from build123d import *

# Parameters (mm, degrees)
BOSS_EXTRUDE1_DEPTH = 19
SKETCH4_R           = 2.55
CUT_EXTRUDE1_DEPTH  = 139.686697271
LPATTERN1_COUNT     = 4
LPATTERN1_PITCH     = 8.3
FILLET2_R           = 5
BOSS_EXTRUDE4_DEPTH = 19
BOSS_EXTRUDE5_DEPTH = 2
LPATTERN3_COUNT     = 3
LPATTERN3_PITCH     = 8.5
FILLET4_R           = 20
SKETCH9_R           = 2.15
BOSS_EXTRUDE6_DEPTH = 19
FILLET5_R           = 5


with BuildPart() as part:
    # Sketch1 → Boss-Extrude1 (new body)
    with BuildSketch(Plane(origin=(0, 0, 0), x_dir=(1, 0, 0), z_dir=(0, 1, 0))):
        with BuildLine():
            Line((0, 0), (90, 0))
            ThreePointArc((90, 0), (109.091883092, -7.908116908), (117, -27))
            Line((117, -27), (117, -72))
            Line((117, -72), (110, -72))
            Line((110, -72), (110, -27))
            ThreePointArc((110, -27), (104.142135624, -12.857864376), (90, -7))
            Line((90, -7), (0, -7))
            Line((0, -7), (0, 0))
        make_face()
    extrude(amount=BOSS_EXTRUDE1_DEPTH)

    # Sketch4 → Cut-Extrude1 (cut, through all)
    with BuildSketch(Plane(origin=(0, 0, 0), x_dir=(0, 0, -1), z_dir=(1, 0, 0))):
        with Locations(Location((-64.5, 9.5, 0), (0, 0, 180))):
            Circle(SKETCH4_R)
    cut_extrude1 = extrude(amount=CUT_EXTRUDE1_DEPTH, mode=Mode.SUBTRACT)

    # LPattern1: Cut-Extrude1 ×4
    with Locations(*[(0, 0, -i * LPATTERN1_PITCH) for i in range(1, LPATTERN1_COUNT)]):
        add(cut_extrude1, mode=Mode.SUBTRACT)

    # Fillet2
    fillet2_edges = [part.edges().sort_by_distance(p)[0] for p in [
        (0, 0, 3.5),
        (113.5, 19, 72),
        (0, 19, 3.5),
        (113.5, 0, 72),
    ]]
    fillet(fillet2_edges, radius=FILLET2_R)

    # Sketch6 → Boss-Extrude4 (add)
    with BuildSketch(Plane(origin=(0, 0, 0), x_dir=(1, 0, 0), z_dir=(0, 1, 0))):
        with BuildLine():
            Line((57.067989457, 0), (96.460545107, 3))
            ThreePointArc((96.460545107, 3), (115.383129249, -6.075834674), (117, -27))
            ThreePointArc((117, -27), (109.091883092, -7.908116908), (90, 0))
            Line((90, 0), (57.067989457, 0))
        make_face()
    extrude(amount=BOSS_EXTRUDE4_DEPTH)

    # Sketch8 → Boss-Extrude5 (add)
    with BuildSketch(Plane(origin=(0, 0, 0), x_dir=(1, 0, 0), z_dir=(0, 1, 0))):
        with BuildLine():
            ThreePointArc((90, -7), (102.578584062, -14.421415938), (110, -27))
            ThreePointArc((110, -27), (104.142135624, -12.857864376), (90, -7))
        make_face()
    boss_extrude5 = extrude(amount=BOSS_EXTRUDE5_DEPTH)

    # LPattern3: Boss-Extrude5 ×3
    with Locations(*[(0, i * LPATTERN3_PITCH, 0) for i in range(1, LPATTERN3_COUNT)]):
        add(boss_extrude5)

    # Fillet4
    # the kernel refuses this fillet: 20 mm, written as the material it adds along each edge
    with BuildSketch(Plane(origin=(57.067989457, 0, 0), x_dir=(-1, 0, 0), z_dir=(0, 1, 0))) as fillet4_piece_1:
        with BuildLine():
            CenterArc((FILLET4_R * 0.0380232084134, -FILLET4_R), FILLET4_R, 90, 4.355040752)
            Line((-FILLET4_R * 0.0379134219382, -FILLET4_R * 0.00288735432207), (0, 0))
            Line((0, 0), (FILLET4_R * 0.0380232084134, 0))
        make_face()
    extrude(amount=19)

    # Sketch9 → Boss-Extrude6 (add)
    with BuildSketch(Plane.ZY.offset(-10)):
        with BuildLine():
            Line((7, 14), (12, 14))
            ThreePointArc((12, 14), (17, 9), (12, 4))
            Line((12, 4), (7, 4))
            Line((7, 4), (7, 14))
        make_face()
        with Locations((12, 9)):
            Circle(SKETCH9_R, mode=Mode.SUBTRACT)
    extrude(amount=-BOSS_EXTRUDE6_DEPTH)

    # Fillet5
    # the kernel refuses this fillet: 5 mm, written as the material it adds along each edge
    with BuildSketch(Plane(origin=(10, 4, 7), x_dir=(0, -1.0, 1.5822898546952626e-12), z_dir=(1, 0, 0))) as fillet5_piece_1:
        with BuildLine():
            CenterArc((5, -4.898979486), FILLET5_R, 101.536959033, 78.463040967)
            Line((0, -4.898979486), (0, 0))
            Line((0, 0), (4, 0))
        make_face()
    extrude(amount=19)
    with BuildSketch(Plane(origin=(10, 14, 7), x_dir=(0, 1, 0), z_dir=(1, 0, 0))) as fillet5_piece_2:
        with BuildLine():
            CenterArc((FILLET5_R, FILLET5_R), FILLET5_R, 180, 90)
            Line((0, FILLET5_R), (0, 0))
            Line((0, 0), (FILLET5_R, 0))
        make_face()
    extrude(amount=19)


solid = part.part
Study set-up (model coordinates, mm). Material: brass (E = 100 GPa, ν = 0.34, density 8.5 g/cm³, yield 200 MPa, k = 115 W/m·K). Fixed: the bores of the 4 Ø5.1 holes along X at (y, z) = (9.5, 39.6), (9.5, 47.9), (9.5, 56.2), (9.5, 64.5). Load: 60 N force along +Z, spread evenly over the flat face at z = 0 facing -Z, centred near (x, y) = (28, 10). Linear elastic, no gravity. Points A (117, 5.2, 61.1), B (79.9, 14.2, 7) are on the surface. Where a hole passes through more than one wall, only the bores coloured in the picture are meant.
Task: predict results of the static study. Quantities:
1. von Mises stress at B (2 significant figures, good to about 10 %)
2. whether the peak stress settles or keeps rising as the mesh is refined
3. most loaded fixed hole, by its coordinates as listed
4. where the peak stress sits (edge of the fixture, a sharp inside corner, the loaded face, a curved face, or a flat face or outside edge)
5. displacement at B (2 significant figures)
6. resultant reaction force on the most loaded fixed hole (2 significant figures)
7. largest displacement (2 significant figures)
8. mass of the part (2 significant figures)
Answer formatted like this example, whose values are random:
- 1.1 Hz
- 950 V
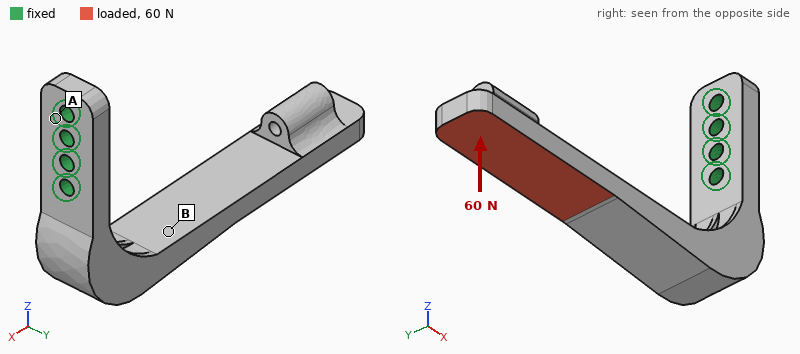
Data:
- 13 MPa
- keeps rising
- (9.5, 39.6)
- edge of the fixture
- 0.074 mm
- 150 N
- 0.33 mm
- 240 g
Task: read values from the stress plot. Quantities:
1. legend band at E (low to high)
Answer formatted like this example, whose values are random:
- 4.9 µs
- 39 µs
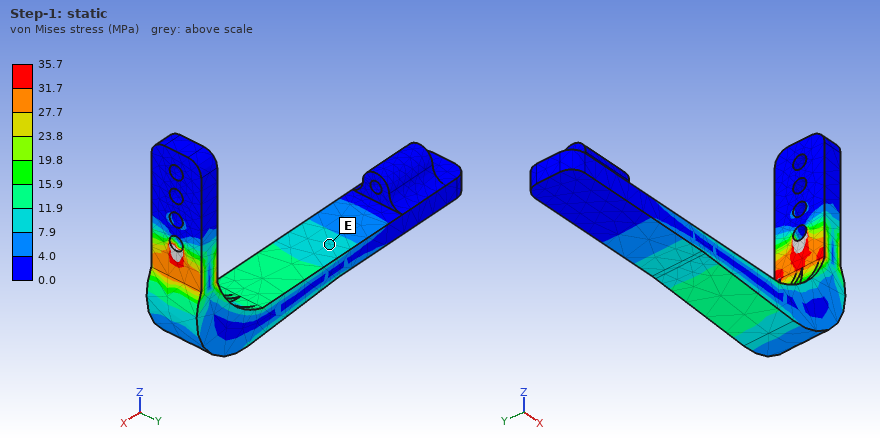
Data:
- 7.9 to 11.9 MPa
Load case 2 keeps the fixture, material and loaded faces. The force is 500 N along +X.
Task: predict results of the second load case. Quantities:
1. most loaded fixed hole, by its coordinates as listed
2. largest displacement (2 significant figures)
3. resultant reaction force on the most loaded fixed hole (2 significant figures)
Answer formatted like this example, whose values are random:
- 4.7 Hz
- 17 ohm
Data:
- (9.5, 39.6)
- 0.66 mm
- 1000 N
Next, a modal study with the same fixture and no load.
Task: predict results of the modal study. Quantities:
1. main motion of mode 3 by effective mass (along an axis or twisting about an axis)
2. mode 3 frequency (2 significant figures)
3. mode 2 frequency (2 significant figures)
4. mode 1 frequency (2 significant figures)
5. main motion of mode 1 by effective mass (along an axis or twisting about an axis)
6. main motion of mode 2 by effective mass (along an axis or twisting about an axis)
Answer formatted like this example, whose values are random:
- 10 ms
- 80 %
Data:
- along X
- 1000 Hz
- 340 Hz
- 260 Hz
- along Z
- along Y
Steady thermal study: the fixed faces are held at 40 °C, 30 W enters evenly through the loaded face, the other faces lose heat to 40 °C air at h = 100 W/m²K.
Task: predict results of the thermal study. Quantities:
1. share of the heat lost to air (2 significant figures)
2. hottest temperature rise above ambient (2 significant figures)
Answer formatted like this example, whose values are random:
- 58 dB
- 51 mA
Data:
- 78 %
- 64 K
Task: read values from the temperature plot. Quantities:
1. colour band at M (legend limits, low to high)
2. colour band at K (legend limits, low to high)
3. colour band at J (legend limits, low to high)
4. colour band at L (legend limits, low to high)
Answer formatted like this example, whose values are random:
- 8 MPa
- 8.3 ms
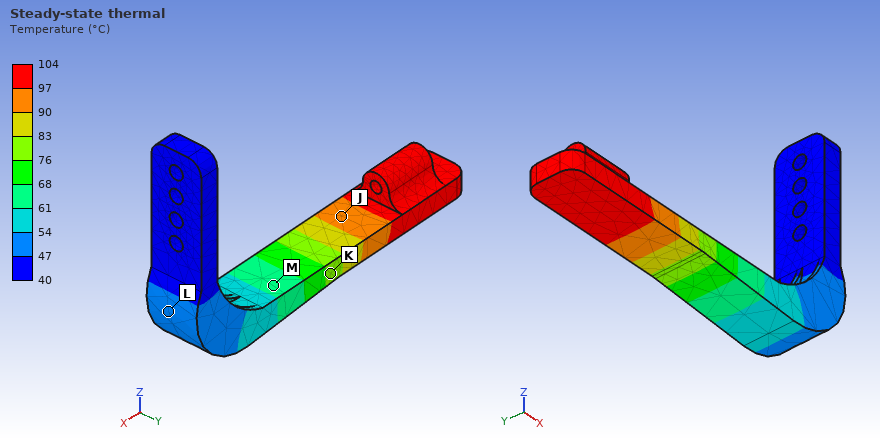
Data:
- 61 to 68 °C
- 76 to 83 °C
- 90 to 97 °C
- 47 to 54 °C
